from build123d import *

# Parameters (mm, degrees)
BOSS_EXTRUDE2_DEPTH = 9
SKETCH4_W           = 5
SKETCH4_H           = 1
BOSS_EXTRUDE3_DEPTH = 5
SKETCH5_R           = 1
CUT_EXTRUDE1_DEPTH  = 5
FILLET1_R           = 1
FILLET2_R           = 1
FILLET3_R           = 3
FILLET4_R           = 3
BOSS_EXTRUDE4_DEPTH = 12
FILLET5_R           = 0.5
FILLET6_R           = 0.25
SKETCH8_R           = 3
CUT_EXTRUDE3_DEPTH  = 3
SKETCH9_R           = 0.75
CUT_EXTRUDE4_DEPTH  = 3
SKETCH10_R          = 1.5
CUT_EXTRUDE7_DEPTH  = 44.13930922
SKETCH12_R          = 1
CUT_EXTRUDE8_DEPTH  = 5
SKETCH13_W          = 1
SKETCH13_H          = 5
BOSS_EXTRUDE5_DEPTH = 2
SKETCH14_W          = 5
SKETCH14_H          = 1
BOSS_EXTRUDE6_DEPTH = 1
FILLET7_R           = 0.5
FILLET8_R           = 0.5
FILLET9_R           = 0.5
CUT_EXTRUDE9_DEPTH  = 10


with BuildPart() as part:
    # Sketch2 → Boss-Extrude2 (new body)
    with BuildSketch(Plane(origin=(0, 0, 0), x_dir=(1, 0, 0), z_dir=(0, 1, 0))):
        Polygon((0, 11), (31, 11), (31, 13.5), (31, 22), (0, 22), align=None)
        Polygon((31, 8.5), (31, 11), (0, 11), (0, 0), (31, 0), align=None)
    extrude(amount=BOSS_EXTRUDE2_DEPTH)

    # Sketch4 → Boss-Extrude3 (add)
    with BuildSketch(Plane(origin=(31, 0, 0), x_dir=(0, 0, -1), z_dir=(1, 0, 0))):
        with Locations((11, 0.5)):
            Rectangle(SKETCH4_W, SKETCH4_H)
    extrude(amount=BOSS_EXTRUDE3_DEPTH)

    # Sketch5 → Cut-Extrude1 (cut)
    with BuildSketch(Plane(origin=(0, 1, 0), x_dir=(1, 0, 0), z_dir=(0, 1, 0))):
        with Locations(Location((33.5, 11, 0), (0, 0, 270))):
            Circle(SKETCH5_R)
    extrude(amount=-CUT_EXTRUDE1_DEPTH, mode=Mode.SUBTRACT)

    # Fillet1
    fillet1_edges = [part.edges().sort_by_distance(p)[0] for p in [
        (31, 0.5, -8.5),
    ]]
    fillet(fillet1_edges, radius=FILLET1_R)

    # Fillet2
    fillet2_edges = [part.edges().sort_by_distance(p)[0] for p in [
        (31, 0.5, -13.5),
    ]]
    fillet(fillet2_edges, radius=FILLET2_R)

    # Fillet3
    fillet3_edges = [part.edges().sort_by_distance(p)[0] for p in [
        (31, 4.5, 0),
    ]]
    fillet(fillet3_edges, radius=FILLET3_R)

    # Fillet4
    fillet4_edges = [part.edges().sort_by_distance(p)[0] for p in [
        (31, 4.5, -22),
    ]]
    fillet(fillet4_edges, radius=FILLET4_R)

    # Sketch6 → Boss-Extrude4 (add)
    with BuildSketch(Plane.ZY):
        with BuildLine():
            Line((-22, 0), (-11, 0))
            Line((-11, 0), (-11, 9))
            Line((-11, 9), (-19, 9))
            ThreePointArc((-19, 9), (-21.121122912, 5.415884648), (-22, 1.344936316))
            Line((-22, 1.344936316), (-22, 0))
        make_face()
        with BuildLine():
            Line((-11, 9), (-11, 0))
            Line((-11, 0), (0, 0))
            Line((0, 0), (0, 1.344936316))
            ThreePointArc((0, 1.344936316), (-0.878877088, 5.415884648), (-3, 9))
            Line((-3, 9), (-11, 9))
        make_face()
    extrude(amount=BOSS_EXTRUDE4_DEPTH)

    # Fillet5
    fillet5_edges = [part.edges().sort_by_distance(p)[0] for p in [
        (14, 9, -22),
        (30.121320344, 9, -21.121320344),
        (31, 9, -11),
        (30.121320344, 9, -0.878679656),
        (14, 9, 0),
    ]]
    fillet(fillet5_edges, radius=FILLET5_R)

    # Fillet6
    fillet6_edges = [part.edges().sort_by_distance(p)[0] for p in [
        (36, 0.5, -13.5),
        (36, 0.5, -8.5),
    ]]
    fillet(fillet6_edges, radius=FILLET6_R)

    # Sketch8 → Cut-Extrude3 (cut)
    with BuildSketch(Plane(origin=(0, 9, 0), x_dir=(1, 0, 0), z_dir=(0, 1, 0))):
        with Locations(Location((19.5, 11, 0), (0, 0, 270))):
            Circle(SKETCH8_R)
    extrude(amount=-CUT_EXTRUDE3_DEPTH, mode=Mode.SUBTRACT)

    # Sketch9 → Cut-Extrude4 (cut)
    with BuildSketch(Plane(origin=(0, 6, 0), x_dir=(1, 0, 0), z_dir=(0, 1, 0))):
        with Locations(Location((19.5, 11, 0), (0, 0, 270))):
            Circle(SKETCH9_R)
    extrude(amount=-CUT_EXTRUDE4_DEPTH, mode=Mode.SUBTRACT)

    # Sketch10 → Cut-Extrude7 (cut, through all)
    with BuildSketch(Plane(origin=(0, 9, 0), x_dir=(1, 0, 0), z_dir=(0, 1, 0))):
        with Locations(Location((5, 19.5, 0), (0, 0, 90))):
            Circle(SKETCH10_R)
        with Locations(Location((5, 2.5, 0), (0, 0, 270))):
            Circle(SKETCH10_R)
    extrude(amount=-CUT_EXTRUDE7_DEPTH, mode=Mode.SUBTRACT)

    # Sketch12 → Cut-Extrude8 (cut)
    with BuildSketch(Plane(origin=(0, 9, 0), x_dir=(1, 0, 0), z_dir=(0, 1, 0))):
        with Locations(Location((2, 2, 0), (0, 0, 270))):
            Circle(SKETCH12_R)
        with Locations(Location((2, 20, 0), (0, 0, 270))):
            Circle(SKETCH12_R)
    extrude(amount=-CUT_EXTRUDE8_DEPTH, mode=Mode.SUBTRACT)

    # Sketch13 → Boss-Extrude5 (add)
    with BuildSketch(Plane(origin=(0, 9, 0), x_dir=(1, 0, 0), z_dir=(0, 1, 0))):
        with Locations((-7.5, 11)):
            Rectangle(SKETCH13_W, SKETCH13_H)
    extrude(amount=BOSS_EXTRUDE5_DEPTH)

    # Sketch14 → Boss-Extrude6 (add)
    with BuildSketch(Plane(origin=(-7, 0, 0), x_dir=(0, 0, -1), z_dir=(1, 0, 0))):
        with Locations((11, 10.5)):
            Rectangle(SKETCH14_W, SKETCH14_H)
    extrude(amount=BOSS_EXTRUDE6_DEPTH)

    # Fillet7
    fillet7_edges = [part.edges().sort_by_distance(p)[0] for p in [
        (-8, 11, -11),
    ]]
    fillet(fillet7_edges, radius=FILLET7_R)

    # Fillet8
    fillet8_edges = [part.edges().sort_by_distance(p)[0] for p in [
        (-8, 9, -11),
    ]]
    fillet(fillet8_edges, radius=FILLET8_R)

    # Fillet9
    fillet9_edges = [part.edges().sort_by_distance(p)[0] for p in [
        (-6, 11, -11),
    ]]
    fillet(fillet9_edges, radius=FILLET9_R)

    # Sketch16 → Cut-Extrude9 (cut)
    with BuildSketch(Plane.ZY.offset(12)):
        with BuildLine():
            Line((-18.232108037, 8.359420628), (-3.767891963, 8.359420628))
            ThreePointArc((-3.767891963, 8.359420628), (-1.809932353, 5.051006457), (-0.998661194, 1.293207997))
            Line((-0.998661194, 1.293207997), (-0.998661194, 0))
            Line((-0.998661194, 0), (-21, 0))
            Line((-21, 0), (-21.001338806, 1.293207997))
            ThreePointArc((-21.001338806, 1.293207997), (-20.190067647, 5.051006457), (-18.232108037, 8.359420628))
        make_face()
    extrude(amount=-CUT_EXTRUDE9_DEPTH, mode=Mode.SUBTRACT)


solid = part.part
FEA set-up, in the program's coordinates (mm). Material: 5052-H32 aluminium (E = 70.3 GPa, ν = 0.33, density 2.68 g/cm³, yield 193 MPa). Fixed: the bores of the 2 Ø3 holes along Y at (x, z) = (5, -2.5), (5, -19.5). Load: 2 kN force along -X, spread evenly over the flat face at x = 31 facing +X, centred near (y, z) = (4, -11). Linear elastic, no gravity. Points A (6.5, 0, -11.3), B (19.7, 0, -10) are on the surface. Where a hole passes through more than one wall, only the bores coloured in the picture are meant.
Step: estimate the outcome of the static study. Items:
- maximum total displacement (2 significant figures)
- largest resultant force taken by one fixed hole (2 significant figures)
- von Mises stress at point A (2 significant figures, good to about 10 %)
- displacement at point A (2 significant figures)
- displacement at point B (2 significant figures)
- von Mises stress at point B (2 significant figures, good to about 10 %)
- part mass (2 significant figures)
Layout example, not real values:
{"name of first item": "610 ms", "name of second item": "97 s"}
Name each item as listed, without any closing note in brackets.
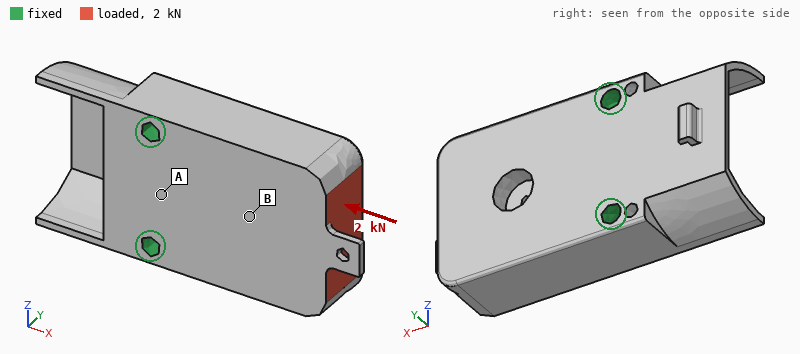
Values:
{"maximum total displacement": "5.1 µm", "largest resultant force taken by one fixed hole": "1.0 kN", "von Mises stress at point A": "3.4 MPa", "displacement at point A": "1.1 µm", "displacement at point B": "2.5 µm", "von Mises stress at point B": "11 MPa", "part mass": "18 g"}
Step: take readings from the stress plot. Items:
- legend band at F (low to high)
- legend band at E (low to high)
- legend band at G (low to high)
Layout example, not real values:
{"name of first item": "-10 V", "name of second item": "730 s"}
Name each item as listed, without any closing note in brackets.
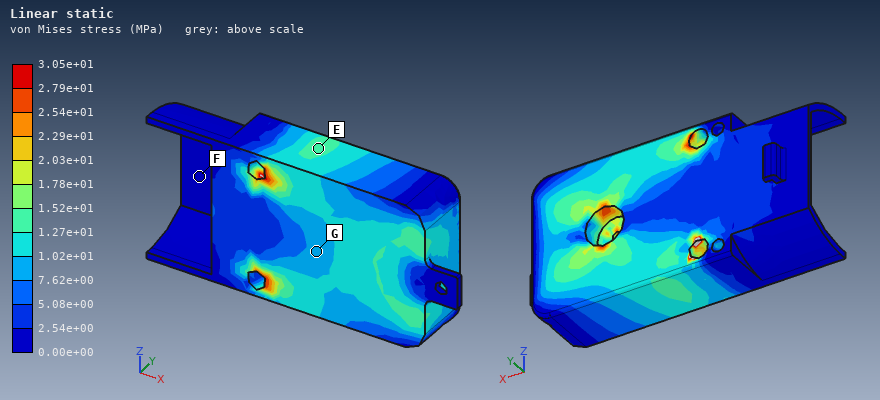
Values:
{"legend band at F": "0.00e+00 to 2.54e+00 MPa", "legend band at E": "1.27e+01 to 1.52e+01 MPa", "legend band at G": "7.62e+00 to 1.02e+01 MPa"}
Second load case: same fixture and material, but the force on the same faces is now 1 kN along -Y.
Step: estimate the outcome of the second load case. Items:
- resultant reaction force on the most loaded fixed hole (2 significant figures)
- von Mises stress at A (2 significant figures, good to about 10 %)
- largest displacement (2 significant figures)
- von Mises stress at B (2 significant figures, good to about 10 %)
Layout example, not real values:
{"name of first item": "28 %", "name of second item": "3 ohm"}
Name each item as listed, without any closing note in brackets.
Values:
{"resultant reaction force on the most loaded fixed hole": "500 N", "von Mises stress at A": "38 MPa", "largest displacement": "0.10 mm", "von Mises stress at B": "41 MPa"}
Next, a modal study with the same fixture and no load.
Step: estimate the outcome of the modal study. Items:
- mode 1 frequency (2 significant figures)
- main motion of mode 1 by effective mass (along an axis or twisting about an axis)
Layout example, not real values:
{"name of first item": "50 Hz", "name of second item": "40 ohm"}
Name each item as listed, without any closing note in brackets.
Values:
{"mode 1 frequency": "9500 Hz", "main motion of mode 1 by effective mass": "along Y"}
